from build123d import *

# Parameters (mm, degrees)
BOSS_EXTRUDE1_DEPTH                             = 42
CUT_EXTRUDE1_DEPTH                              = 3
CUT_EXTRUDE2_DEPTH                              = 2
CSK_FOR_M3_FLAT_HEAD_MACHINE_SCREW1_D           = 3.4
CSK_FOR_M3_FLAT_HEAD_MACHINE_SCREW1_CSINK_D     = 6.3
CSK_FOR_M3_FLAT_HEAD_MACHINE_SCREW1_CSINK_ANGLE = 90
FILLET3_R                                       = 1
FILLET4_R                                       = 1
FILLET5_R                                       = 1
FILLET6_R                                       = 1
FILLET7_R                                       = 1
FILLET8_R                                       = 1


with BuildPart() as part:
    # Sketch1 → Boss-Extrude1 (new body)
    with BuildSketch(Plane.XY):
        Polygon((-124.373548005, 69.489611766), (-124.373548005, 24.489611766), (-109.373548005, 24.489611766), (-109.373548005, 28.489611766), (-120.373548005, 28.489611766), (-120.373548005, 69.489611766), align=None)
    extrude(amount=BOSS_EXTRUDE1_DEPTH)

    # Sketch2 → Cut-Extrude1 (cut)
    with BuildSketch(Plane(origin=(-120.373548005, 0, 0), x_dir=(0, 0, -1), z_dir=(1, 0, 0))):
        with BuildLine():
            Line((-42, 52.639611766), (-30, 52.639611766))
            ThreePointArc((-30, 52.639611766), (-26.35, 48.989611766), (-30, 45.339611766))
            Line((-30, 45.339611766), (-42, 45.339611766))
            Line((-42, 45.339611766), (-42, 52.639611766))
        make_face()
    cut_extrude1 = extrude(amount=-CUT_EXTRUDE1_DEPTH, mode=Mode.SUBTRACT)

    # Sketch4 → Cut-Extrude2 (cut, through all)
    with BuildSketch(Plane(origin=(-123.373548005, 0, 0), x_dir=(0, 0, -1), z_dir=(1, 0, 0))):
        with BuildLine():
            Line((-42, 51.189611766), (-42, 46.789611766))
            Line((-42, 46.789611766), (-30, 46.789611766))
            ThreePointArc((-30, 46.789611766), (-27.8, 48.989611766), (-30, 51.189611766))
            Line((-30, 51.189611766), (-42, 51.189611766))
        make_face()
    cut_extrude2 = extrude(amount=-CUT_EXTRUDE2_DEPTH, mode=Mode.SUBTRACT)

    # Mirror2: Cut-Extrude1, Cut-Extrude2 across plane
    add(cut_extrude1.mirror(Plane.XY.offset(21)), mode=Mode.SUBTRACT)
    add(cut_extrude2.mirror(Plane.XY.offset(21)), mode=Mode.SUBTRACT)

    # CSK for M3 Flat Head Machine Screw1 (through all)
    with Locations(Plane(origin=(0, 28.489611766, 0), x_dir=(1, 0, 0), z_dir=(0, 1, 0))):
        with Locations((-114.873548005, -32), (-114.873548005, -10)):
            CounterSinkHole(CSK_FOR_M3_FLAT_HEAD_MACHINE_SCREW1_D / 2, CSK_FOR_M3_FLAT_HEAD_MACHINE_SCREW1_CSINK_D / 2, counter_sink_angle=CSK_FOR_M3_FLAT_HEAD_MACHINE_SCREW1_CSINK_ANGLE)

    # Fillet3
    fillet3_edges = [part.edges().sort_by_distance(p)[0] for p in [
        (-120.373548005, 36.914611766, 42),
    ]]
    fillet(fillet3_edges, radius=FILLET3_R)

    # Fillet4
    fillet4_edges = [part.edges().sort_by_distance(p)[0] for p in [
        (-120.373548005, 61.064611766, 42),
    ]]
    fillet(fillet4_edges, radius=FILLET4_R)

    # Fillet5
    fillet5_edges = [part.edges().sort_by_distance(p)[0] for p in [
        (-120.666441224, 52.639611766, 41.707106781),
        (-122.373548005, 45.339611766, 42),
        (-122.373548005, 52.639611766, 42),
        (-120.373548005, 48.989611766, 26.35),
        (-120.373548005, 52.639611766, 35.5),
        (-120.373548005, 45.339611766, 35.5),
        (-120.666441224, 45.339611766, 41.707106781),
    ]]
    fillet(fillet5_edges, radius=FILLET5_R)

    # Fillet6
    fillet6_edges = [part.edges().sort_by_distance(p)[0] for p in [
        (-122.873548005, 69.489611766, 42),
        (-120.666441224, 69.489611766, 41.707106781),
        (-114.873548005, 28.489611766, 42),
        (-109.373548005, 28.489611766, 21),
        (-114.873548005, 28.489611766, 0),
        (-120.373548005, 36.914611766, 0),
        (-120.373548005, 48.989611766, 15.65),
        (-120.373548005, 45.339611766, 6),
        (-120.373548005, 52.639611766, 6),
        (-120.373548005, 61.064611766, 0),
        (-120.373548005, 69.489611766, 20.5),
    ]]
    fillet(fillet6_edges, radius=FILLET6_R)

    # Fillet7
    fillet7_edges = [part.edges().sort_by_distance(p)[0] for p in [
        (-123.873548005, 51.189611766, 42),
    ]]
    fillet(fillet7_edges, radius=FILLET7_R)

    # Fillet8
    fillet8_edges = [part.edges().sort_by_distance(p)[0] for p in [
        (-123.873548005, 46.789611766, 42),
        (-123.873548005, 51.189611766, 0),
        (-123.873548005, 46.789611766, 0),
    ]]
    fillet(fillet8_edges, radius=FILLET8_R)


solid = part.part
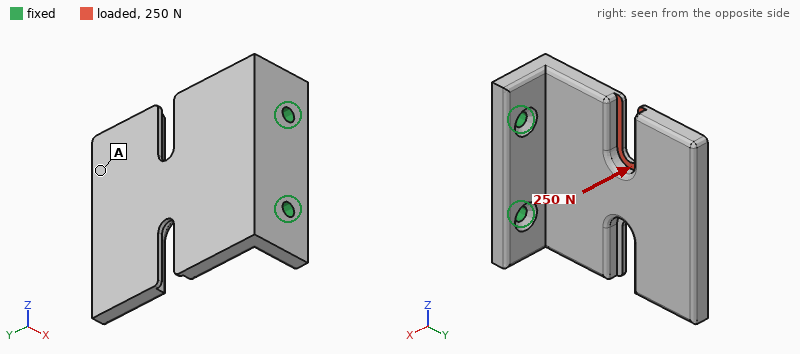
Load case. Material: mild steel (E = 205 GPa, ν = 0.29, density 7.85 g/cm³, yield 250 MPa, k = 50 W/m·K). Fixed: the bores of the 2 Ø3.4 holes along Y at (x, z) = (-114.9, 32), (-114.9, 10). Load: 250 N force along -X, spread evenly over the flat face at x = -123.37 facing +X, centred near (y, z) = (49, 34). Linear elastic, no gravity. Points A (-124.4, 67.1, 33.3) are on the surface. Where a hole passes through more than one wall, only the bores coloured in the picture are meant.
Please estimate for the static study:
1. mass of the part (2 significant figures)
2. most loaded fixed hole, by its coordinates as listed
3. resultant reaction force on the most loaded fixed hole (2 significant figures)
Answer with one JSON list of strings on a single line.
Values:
["67 g", "(-114.9, 32)", "260 N"]
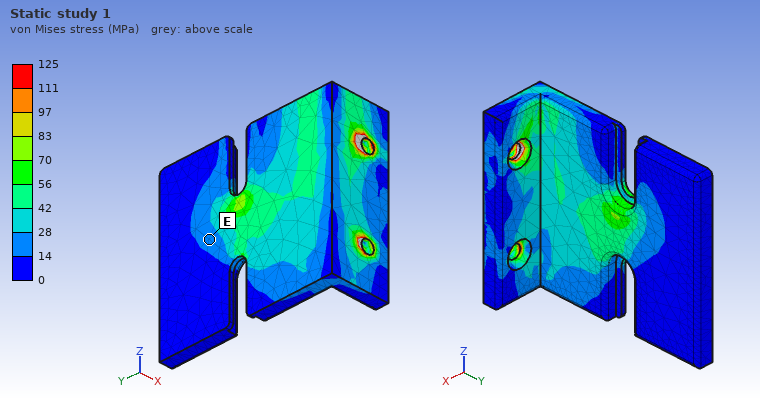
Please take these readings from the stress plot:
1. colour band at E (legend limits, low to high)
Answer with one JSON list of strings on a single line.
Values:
["14 to 28 MPa"]
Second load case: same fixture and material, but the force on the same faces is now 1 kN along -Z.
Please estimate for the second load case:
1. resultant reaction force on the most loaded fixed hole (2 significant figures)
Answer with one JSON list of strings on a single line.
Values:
["1.1 kN"]
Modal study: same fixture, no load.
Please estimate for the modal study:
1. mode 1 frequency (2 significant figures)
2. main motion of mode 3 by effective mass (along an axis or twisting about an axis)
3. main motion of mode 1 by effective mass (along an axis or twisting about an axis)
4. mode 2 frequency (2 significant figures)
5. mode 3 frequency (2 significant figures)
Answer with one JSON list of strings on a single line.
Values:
["1200 Hz", "along Z", "along X", "2600 Hz", "3800 Hz"]
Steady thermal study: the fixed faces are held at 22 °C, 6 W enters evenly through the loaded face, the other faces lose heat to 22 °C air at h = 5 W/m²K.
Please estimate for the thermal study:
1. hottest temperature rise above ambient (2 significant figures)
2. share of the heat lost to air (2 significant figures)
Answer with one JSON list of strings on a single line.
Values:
["48 K", "7.9 %"]
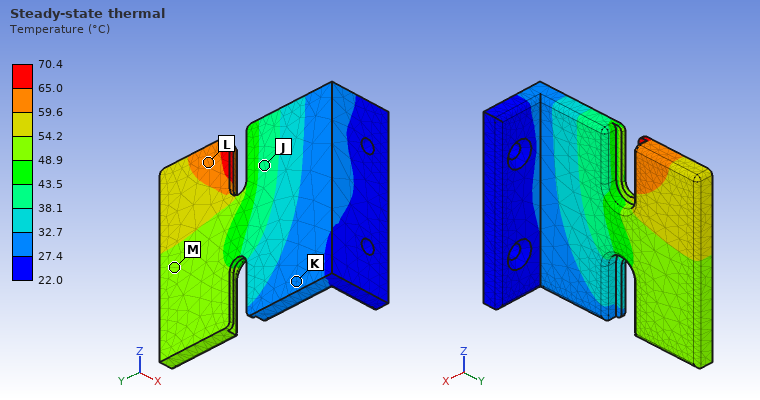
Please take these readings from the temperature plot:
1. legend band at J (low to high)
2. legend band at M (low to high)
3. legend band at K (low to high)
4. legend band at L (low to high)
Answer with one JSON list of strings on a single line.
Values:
["38.1 to 43.5 °C", "48.9 to 54.2 °C", "27.4 to 32.7 °C", "59.6 to 65.0 °C"]
